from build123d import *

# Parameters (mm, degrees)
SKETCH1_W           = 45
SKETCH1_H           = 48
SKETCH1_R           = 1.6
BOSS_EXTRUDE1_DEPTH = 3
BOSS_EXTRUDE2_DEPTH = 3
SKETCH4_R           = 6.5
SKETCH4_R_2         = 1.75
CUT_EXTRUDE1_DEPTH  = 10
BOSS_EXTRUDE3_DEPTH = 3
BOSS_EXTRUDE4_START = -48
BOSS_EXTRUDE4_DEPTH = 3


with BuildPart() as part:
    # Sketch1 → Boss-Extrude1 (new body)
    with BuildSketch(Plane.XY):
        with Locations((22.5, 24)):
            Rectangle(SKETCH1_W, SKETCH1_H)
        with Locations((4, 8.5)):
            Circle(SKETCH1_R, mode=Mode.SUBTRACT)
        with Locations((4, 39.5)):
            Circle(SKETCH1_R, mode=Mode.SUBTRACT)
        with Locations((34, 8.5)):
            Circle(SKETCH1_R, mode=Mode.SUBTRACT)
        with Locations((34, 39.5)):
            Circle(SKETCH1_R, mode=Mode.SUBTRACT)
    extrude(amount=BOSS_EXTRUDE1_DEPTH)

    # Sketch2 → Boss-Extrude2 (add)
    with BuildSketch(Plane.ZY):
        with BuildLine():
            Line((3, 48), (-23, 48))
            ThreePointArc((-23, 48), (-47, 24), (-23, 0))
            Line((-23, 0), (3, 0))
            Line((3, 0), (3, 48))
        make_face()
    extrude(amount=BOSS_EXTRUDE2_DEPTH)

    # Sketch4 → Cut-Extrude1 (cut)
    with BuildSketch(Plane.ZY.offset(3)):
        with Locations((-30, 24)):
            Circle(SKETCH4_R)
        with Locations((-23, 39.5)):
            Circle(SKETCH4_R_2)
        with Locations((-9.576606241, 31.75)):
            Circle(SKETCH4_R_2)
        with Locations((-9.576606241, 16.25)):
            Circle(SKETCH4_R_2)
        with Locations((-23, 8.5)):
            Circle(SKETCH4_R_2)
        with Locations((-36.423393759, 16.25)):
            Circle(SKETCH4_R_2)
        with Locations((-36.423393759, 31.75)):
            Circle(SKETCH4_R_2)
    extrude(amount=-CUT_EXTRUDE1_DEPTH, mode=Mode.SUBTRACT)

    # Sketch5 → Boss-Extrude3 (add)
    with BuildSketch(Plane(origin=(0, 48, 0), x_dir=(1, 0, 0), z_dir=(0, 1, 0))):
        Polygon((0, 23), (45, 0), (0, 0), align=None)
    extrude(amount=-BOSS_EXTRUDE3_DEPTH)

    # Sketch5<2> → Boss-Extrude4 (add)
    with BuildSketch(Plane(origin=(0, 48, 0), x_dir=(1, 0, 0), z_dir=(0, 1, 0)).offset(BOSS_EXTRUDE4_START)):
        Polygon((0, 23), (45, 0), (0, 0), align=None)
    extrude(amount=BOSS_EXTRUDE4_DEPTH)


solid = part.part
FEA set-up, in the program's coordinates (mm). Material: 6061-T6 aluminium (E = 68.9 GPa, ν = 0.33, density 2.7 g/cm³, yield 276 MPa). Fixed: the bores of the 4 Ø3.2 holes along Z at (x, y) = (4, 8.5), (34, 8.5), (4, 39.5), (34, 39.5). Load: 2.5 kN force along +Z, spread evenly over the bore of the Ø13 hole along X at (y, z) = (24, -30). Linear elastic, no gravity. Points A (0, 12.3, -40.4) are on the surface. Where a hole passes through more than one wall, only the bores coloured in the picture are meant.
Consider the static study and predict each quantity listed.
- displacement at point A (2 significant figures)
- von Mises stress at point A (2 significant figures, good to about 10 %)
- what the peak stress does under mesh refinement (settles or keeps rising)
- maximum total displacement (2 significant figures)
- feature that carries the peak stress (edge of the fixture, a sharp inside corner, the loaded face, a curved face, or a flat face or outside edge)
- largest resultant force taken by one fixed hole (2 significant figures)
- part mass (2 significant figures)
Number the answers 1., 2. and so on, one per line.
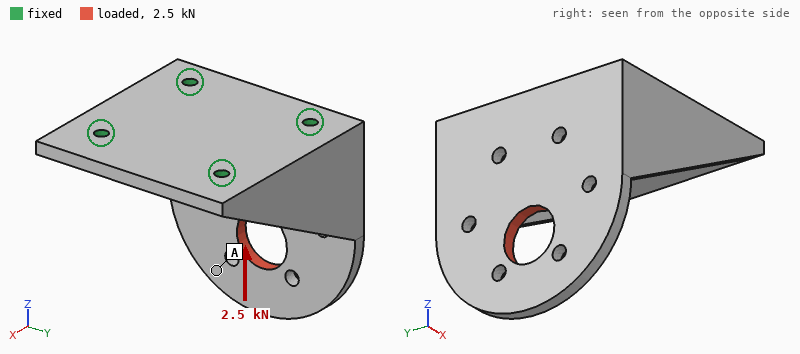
1. 55 µm
2. 15 MPa
3. keeps rising
4. 67 µm
5. edge of the fixture
6. 1.4 kN
7. 42 g
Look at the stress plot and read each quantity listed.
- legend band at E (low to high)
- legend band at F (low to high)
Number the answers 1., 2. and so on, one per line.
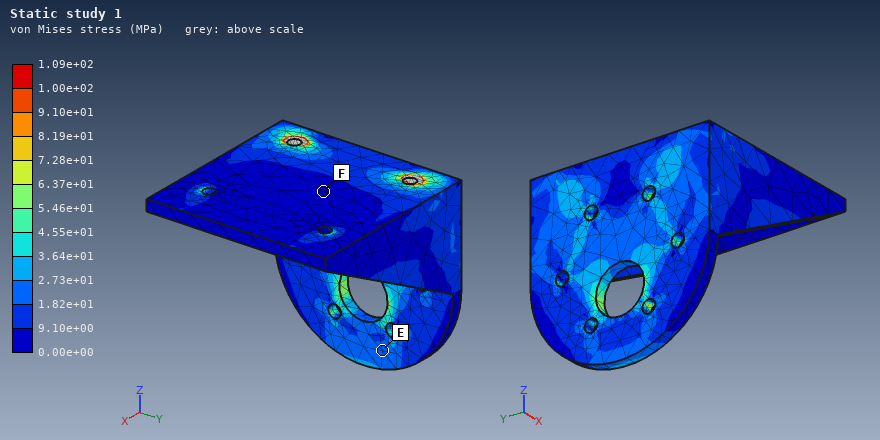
1. 1.82e+01 to 2.73e+01 MPa
2. 0.00e+00 to 9.10e+00 MPa
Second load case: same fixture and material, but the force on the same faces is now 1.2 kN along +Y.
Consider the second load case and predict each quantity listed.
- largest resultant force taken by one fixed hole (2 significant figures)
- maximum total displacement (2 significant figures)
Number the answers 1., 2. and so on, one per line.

1. 1.3 kN
2. 75 µm
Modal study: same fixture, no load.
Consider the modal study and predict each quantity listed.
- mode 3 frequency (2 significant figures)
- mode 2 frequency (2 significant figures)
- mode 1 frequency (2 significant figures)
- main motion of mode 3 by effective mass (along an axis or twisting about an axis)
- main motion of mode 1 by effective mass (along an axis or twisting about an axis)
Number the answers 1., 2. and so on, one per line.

1. 7500 Hz
2. 6100 Hz
3. 2500 Hz
4. along Y
5. along X
